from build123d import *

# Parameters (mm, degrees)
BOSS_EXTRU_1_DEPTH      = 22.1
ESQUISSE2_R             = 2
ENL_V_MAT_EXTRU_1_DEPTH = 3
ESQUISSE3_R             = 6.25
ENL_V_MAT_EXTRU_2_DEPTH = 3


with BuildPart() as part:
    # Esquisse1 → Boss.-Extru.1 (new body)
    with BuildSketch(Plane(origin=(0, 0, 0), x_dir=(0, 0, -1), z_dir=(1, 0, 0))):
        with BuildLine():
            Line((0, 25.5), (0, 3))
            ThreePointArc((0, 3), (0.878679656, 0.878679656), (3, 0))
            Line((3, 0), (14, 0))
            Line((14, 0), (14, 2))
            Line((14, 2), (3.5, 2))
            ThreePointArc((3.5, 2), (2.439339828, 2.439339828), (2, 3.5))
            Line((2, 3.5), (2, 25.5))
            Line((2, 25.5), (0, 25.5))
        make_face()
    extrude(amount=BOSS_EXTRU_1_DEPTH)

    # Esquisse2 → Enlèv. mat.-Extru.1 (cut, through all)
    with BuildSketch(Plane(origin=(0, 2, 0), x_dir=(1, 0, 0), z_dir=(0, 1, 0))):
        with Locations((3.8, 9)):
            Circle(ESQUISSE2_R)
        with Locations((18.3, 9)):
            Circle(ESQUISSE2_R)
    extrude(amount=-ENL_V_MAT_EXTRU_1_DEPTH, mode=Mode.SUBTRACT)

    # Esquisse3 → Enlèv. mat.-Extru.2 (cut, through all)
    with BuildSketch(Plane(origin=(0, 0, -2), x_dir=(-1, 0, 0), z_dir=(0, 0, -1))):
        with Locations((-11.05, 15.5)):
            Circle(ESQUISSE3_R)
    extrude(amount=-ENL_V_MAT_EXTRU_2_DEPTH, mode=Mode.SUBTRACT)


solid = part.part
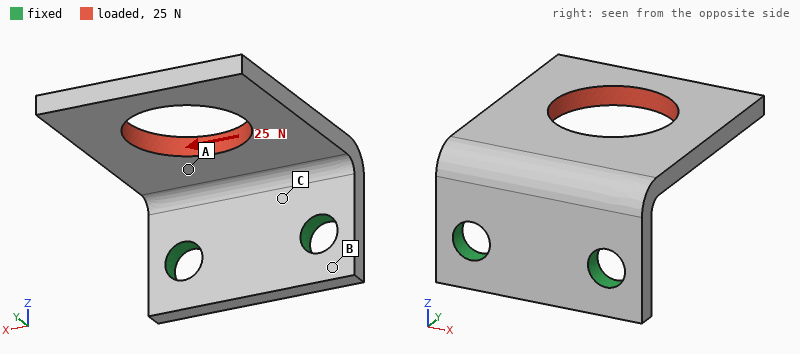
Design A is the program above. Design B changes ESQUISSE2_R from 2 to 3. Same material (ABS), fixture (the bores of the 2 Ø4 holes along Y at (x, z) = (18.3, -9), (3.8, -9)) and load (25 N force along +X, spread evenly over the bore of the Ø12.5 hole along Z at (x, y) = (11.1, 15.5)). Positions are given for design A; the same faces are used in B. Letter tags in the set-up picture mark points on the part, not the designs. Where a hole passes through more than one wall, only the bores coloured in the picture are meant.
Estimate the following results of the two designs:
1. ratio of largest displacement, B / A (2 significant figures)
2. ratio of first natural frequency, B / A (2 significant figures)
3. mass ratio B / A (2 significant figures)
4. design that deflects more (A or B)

0.73
1.1
0.95
A
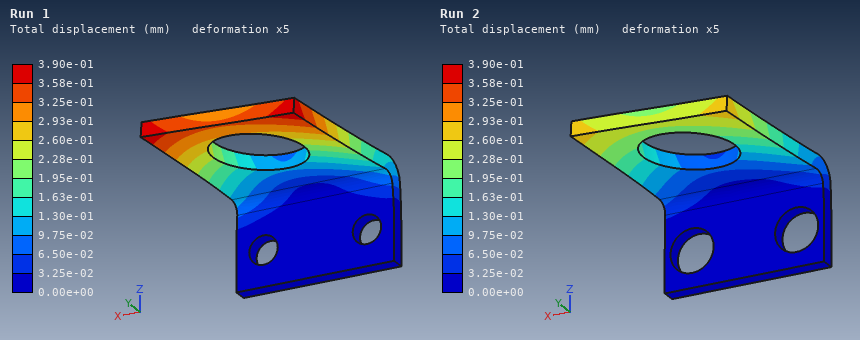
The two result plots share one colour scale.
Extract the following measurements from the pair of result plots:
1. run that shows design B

Run 2
